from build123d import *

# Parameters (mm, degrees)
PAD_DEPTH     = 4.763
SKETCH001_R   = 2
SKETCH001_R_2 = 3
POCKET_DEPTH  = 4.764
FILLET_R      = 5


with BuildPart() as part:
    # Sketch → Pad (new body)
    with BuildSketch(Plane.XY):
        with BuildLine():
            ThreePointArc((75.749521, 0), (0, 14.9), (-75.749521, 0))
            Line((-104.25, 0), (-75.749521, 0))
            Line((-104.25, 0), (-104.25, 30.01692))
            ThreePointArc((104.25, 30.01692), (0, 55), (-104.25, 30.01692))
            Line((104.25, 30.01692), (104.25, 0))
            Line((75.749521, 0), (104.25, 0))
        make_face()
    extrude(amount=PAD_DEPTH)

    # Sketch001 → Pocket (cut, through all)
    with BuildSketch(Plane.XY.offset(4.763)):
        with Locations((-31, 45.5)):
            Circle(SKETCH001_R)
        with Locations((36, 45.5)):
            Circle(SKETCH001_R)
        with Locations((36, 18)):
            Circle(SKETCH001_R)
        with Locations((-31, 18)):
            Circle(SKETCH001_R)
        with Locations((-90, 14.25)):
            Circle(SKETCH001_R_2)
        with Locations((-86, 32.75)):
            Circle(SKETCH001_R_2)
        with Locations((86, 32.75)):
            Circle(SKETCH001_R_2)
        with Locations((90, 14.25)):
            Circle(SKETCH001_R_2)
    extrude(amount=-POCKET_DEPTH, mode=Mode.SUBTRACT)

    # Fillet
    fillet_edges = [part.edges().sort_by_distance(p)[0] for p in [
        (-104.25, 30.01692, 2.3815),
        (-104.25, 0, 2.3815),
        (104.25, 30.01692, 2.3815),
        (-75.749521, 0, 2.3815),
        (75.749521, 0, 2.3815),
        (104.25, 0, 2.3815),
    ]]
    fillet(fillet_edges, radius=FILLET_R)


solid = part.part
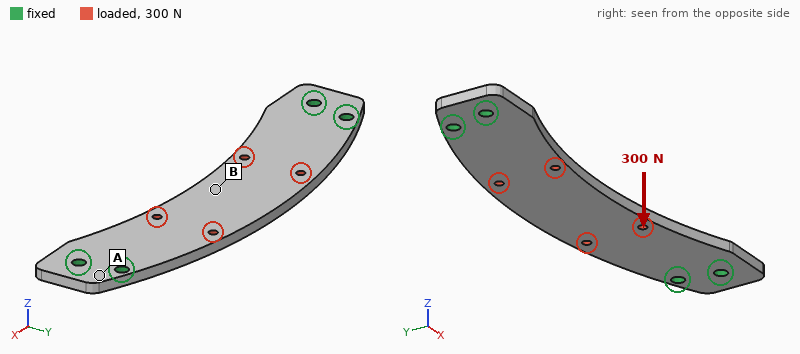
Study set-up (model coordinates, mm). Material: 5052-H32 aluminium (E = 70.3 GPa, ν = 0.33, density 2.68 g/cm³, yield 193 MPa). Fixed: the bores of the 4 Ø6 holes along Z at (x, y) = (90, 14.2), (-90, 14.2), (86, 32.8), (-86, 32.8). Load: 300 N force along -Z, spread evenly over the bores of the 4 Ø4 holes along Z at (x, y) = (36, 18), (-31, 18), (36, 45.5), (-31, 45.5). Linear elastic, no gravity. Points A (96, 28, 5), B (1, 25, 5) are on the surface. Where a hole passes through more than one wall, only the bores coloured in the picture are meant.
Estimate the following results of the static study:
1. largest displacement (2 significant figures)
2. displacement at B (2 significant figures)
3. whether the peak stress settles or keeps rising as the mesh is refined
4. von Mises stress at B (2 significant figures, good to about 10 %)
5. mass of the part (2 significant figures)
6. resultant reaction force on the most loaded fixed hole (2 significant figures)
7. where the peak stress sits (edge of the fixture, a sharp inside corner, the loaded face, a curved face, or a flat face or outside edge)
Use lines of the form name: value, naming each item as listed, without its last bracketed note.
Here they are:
largest displacement: 0.24 mm
displacement at B: 0.21 mm
whether the peak stress settles or keeps rising as the mesh is refined: keeps rising
von Mises stress at B: 16 MPa
mass of the part: 100 g
resultant reaction force on the most loaded fixed hole: 170 N
where the peak stress sits: edge of the fixture
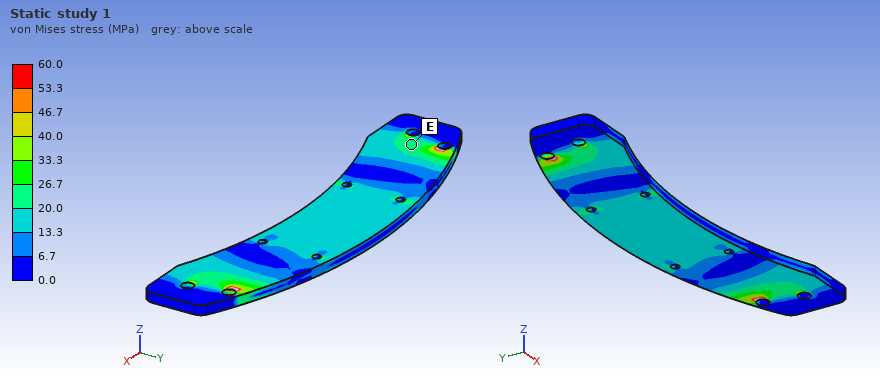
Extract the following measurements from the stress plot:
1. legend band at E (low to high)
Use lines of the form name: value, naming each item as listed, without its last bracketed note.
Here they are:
legend band at E: 20.0 to 26.7 MPa
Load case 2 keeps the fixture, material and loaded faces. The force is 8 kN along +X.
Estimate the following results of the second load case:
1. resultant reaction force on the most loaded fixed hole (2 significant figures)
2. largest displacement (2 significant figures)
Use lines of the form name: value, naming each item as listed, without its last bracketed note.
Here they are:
resultant reaction force on the most loaded fixed hole: 2.4 kN
largest displacement: 21 µm
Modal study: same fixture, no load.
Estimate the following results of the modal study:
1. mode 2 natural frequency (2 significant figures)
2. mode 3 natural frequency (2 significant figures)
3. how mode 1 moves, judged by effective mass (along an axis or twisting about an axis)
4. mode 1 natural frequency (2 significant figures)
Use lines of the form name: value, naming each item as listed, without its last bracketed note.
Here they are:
mode 2 natural frequency: 2300 Hz
mode 3 natural frequency: 2300 Hz
how mode 1 moves, judged by effective mass: along Z
mode 1 natural frequency: 830 Hz
